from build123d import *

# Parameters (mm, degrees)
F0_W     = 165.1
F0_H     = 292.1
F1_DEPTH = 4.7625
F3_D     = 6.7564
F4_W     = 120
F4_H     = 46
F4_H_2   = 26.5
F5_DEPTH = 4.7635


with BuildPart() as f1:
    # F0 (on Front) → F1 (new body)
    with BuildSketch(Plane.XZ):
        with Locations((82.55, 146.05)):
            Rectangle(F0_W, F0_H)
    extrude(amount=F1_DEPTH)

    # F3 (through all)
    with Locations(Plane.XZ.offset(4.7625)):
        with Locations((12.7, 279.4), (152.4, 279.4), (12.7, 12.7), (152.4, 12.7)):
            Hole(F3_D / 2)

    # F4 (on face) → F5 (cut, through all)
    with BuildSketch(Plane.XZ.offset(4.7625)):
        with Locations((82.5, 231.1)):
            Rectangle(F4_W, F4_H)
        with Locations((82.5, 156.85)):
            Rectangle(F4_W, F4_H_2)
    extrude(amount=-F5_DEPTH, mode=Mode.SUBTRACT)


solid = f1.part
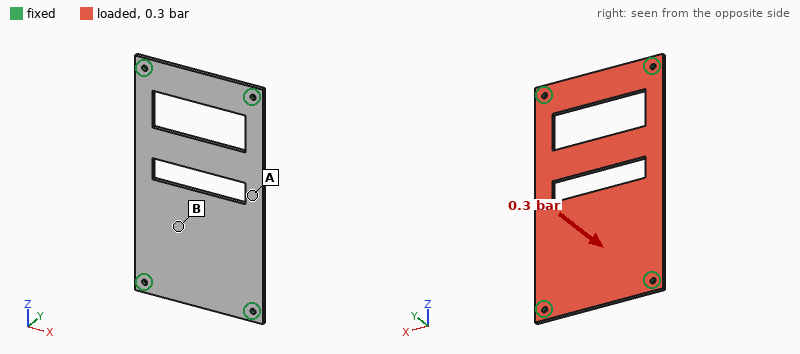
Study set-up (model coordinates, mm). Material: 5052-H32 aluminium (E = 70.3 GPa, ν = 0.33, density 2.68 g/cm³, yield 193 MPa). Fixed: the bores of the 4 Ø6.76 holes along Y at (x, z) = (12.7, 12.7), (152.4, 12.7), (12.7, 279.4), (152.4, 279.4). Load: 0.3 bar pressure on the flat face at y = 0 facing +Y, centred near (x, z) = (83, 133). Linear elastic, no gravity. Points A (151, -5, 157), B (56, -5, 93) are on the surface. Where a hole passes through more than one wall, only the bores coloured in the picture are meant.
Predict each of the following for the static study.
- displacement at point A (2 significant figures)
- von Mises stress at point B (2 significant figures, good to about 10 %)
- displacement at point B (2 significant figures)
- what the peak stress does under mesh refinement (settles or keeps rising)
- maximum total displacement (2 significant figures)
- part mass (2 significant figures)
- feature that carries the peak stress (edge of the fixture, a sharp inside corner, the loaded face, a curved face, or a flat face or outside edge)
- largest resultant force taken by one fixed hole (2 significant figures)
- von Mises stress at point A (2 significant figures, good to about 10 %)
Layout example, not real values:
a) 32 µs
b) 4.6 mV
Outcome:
a) 1.2 mm
b) 8.4 MPa
c) 0.82 mm
d) keeps rising
e) 1.3 mm
f) 500 g
g) edge of the fixture
h) 340 N
i) 61 MPa
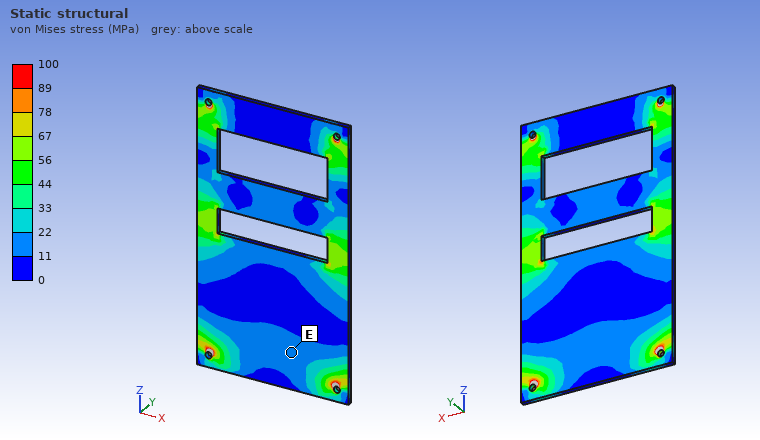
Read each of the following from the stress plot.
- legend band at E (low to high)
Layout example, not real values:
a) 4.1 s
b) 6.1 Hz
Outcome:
a) 11 to 22 MPa
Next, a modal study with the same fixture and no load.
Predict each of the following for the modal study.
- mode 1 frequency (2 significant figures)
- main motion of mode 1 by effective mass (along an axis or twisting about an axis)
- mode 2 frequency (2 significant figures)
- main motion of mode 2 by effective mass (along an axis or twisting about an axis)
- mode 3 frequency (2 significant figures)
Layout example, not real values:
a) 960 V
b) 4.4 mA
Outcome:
a) 260 Hz
b) along Y
c) 480 Hz
d) twisting about Z
e) 660 Hz
